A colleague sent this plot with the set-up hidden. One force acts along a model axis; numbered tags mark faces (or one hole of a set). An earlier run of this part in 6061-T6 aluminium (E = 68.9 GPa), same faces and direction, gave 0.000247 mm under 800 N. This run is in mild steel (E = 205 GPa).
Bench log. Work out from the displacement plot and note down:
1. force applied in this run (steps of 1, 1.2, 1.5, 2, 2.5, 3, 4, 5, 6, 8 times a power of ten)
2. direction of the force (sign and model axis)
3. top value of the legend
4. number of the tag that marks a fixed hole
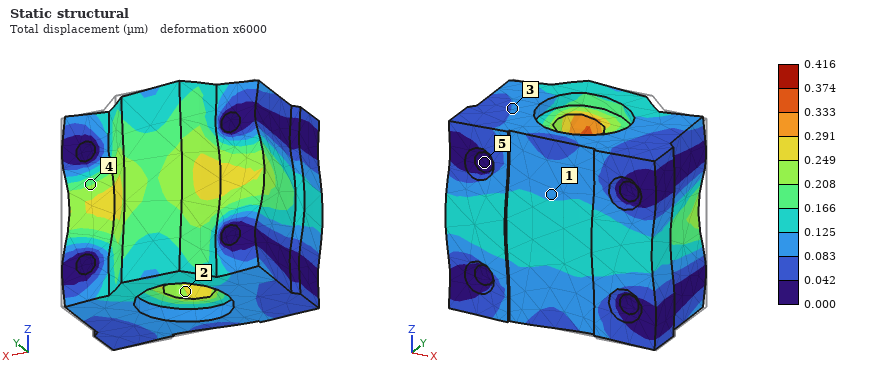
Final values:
4 kN
-X
0.416 µm
5
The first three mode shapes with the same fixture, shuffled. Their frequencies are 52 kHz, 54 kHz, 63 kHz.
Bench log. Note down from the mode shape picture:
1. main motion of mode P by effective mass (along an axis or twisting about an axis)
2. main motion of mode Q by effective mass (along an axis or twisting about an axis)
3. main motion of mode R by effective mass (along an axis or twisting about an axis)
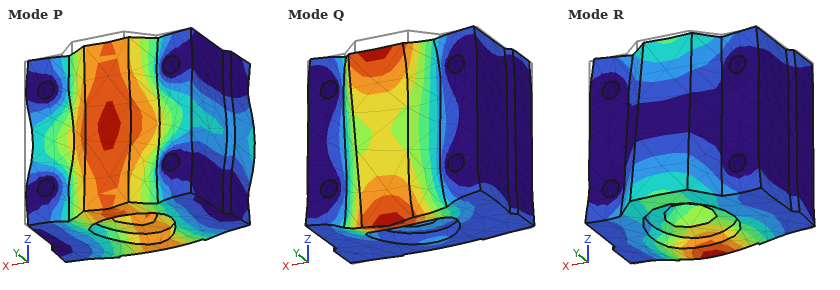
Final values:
along Y
along Z
along Z
